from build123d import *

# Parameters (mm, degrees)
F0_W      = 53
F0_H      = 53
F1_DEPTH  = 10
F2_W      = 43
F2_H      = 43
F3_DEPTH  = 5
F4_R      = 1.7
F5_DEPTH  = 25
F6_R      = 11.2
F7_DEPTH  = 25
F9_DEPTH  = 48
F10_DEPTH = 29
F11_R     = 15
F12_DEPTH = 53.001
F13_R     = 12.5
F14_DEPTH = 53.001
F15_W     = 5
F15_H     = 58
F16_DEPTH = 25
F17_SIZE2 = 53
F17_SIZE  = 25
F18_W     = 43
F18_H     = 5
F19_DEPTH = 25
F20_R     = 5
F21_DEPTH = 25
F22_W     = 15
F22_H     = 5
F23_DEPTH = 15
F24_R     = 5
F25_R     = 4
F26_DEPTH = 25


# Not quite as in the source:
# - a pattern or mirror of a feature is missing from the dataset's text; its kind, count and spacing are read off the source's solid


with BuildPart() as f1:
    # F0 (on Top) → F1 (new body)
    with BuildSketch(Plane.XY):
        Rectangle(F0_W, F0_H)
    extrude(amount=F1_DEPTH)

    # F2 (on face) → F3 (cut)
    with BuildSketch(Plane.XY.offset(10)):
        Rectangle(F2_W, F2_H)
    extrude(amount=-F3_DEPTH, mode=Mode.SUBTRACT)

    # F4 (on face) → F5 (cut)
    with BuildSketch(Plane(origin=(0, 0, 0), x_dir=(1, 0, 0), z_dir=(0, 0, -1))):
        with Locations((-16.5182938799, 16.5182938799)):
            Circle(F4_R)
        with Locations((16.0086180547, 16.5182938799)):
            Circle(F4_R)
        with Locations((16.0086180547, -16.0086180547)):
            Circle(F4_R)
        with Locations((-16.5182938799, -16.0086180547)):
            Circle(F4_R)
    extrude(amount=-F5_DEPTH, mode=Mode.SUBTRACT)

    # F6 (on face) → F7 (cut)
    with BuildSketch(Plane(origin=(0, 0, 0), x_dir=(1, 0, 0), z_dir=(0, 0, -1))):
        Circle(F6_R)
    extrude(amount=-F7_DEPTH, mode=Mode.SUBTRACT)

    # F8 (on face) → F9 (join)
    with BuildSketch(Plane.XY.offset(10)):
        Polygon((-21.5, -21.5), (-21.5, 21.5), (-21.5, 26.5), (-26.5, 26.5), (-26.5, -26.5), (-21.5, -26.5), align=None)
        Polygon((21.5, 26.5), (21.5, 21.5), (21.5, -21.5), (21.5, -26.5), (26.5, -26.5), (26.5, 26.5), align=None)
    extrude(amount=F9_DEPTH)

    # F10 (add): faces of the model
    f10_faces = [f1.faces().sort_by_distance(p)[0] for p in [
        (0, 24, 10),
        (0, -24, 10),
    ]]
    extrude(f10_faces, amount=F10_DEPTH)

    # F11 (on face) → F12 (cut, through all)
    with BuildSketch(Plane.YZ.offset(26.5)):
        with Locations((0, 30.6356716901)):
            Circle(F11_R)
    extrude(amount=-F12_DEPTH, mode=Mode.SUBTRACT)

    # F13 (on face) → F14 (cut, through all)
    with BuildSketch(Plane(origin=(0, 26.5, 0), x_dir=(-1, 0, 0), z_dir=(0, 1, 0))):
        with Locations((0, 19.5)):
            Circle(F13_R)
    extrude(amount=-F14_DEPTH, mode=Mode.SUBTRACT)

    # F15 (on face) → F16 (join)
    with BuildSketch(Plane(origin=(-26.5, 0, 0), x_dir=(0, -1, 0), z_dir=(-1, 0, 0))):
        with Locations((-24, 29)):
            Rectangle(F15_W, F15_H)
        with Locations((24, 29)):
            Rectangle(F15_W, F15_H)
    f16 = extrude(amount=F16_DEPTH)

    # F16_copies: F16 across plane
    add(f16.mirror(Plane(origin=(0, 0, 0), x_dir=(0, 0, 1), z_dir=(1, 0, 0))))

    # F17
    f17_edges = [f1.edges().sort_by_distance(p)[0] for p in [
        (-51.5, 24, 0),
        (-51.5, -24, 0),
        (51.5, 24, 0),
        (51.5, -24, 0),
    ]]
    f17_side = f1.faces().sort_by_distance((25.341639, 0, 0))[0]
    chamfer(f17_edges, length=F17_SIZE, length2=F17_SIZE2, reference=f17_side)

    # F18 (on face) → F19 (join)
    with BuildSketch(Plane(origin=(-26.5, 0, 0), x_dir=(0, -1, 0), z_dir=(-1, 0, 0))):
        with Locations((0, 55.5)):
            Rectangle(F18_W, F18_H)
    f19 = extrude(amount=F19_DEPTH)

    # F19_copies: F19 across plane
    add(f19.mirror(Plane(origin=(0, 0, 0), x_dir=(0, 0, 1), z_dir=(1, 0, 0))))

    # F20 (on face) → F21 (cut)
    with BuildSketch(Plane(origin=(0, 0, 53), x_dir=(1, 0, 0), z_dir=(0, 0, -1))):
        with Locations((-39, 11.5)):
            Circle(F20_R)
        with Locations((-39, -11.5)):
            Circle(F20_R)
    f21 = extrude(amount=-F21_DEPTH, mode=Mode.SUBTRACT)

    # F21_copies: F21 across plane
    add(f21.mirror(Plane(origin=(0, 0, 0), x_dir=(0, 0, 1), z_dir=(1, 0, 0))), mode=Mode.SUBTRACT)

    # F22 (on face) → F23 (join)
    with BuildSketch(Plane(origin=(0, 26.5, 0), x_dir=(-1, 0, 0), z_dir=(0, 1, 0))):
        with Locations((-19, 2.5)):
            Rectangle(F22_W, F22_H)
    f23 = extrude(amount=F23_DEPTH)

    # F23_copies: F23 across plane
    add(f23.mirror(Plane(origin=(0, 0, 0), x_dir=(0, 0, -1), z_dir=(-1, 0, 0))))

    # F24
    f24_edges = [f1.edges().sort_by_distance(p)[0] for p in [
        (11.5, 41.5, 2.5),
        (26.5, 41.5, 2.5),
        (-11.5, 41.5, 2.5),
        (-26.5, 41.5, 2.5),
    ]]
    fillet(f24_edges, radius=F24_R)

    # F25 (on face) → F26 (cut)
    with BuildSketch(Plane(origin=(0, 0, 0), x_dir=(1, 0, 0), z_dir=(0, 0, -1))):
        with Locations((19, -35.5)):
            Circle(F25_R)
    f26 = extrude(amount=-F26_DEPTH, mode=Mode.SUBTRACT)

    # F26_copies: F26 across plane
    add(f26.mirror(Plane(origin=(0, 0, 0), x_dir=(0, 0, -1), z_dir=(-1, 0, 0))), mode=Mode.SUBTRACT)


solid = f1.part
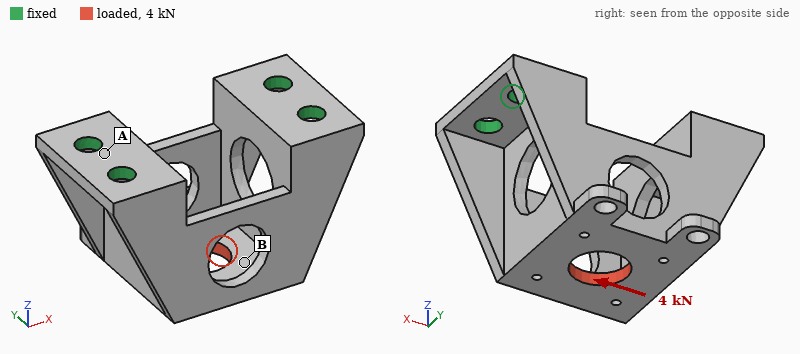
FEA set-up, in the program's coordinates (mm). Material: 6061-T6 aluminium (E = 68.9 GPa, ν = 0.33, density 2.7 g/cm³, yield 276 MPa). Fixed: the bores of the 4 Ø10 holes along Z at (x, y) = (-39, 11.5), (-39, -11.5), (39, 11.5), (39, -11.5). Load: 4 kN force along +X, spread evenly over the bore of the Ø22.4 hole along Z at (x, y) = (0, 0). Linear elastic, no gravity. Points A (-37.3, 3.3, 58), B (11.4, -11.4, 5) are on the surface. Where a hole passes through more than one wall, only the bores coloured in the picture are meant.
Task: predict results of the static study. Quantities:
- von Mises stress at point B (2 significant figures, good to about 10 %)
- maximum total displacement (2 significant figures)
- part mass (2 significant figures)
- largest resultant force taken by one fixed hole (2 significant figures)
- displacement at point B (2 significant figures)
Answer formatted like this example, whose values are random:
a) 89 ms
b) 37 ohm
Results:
a) 22 MPa
b) 76 µm
c) 190 g
d) 1.6 kN
e) 72 µm
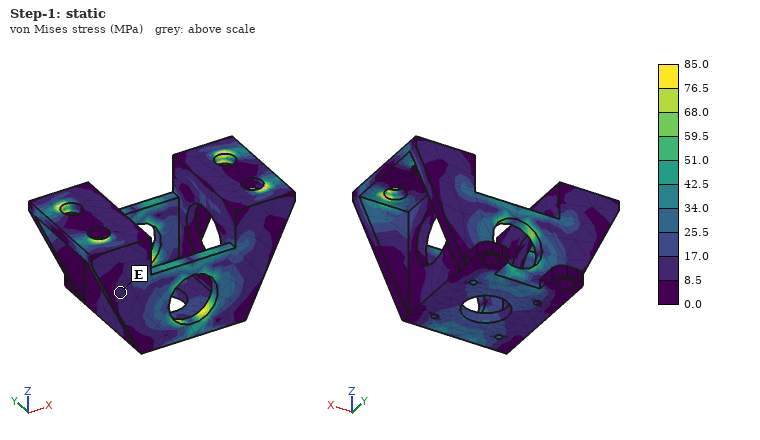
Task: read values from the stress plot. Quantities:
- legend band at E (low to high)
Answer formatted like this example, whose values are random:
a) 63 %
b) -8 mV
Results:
a) 8.5 to 17.0 MPa
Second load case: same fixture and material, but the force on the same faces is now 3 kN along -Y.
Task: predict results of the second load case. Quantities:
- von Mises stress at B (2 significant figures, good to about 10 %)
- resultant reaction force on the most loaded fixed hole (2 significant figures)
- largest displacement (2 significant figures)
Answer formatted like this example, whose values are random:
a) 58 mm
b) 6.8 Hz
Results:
a) 11 MPa
b) 2.6 kN
c) 0.13 mm
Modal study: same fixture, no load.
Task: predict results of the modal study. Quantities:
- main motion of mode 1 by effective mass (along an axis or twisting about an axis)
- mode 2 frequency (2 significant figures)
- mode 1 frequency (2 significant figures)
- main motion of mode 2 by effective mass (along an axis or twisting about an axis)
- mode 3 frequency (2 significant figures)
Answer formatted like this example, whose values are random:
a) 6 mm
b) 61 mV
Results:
a) along Y
b) 4100 Hz
c) 2800 Hz
d) along X
e) 4600 Hz
